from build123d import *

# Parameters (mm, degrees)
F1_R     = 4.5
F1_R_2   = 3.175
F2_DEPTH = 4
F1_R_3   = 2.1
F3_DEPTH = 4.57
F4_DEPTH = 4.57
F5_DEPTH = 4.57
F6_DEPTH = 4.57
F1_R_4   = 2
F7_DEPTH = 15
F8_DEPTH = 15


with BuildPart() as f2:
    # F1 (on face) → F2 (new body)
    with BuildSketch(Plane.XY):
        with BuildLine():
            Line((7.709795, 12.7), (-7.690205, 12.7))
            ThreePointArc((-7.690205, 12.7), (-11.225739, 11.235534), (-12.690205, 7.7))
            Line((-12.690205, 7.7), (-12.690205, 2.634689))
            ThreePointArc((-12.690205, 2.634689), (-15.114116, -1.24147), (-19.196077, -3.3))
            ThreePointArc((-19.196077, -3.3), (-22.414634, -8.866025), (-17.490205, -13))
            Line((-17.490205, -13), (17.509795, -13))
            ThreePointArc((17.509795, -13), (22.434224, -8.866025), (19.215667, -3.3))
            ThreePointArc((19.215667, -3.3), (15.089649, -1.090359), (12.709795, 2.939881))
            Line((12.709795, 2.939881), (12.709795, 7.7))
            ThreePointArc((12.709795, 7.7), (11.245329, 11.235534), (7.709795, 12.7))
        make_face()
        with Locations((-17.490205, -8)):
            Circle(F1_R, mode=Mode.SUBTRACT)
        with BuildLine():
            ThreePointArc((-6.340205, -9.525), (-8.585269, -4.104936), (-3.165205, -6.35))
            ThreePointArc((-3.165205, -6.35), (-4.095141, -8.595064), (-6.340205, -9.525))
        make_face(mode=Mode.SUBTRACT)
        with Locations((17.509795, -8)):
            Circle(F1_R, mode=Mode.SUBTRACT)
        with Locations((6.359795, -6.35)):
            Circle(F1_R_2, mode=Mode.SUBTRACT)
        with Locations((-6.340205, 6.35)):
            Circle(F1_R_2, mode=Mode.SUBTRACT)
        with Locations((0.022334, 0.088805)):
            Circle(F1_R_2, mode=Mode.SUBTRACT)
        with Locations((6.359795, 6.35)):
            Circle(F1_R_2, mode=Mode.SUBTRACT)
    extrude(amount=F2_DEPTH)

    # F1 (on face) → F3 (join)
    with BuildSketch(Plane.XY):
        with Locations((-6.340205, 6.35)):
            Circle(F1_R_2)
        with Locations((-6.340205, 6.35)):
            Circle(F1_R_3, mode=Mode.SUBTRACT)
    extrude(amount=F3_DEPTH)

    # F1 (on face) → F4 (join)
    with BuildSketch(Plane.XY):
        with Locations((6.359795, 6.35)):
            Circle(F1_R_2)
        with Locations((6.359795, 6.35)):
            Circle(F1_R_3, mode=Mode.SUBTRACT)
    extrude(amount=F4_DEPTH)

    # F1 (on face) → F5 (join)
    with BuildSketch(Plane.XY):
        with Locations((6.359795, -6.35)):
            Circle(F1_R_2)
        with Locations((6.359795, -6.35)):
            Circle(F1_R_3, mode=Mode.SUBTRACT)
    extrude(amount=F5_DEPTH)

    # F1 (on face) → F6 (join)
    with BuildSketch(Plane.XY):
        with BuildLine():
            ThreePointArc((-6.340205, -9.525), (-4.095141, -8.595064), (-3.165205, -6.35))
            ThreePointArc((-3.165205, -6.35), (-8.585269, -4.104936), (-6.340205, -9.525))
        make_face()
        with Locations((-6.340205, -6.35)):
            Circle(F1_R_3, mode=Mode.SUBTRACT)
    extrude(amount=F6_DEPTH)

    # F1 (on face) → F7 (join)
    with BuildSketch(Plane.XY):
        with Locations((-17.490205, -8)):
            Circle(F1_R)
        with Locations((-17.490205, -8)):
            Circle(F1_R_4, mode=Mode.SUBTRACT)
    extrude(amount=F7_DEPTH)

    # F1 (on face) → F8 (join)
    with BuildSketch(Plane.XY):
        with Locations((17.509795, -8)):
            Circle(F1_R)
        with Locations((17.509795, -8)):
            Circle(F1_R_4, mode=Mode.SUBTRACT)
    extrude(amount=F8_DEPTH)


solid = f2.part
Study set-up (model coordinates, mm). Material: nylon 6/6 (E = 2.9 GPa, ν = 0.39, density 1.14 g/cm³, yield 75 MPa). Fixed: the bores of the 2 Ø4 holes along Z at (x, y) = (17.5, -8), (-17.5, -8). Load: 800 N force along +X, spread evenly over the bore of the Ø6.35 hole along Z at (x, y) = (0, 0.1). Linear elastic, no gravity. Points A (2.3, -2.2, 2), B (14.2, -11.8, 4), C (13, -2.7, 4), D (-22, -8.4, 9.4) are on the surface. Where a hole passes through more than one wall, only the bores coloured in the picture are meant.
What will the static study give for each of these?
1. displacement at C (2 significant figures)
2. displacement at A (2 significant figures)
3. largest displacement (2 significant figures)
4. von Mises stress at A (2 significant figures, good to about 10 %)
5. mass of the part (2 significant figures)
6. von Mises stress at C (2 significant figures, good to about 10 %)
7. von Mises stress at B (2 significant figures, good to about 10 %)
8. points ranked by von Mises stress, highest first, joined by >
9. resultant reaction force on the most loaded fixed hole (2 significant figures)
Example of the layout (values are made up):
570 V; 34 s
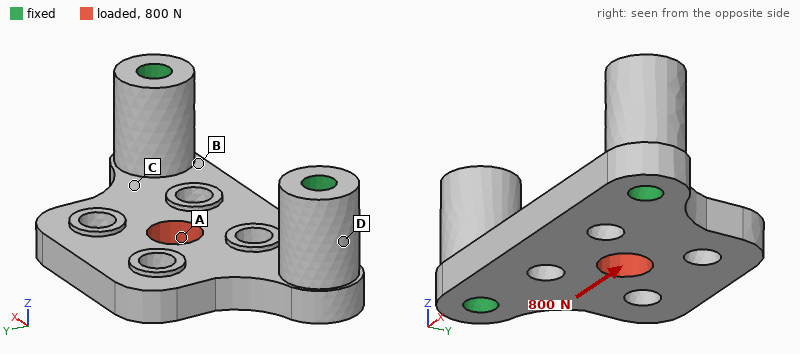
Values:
30 µm; 68 µm; 98 µm; 17 MPa; 4.6 g; 14 MPa; 4.0 MPa; A > C > B > D; 440 N
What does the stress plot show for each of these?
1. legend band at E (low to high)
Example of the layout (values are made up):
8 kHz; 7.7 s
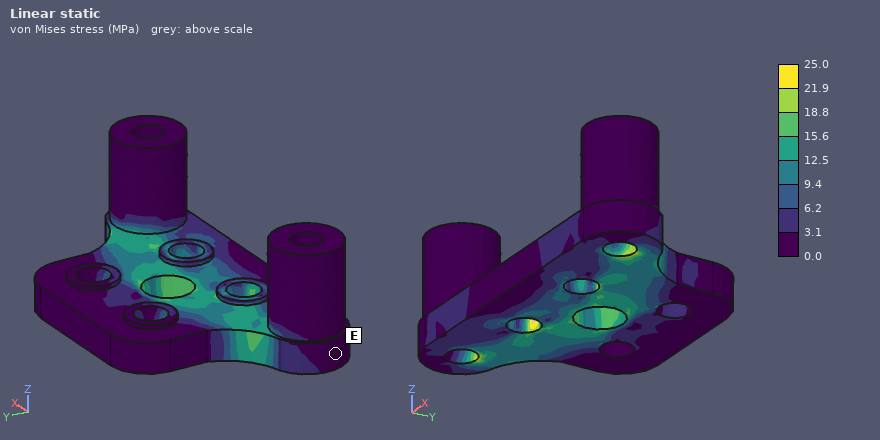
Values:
0.0 to 3.1 MPa
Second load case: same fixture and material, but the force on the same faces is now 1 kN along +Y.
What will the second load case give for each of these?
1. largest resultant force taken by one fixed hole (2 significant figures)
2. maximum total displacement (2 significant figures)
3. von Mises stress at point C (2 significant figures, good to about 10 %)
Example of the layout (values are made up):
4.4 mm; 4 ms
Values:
550 N; 0.20 mm; 17 MPa
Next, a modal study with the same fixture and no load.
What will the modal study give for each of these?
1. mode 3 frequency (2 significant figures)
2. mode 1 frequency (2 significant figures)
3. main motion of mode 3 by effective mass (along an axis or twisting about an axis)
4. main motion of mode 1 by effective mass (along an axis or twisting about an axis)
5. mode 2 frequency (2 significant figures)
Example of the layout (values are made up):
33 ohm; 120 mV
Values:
6500 Hz; 2100 Hz; along Z; along Z; 5300 Hz
